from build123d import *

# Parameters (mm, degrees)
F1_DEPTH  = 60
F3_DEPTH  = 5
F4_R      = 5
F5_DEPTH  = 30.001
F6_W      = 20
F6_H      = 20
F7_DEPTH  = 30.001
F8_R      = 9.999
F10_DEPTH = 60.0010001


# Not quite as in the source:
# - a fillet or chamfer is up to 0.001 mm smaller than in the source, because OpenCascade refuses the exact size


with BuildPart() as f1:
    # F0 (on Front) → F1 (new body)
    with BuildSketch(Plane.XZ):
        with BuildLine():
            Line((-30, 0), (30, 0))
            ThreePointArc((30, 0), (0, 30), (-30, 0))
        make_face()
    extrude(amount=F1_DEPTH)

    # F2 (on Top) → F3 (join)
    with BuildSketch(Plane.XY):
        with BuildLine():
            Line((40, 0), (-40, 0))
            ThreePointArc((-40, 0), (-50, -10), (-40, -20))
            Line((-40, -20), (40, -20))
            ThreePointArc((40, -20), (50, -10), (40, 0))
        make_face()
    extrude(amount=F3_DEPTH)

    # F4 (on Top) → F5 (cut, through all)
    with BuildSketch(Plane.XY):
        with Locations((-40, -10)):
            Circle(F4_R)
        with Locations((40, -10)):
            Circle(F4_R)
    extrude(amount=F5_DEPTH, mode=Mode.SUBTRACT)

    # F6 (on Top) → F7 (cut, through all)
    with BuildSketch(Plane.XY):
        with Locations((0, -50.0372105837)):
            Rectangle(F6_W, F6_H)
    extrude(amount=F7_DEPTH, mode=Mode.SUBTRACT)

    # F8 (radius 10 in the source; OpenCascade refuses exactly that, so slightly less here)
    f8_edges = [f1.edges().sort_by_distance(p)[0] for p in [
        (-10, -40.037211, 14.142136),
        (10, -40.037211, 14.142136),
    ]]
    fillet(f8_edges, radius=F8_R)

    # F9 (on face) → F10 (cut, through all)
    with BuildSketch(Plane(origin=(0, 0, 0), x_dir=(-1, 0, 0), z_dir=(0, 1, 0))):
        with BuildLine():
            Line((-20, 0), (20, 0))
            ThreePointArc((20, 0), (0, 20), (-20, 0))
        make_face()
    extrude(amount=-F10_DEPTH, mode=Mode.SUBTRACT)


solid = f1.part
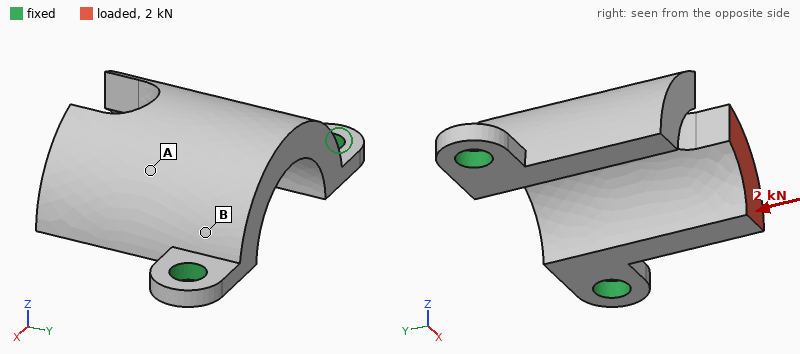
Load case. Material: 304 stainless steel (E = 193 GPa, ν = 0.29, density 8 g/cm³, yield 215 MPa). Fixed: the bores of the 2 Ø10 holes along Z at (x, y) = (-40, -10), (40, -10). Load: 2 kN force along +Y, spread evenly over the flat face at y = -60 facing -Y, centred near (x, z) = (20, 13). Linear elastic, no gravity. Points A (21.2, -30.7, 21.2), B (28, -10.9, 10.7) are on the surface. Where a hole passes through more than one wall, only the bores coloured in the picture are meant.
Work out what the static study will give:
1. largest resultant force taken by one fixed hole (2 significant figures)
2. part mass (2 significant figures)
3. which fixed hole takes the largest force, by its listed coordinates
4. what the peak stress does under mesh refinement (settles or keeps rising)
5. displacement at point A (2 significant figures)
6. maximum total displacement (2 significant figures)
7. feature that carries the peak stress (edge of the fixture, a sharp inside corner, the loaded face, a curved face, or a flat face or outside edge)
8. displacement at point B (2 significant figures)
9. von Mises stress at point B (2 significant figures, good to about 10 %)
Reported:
1.6 kN
370 g
(40, -10)
keeps rising
34 µm
67 µm
edge of the fixture
13 µm
30 MPa
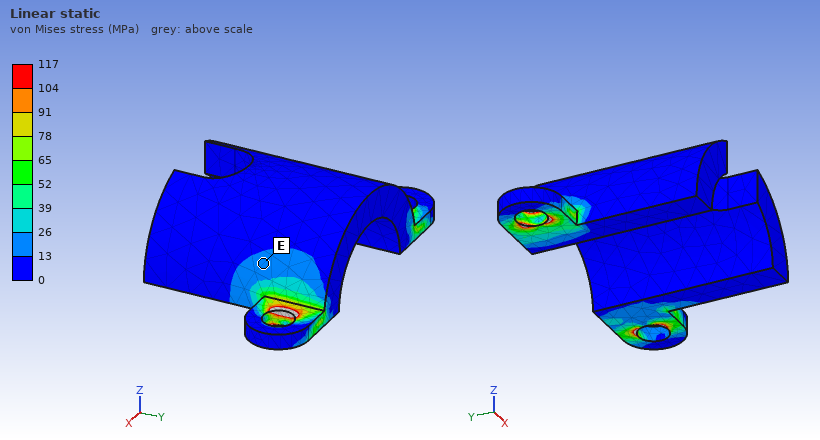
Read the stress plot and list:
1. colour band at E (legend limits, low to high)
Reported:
13 to 26 MPa
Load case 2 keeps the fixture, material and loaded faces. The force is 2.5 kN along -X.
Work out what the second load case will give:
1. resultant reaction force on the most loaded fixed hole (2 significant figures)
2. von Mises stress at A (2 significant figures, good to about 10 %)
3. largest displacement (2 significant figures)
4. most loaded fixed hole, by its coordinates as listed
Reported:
2.2 kN
72 MPa
95 µm
(40, -10)
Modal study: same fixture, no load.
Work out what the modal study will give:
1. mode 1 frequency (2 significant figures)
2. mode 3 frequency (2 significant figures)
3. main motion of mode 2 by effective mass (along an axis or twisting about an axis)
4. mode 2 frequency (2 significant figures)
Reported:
1300 Hz
5900 Hz
along X
3600 Hz
